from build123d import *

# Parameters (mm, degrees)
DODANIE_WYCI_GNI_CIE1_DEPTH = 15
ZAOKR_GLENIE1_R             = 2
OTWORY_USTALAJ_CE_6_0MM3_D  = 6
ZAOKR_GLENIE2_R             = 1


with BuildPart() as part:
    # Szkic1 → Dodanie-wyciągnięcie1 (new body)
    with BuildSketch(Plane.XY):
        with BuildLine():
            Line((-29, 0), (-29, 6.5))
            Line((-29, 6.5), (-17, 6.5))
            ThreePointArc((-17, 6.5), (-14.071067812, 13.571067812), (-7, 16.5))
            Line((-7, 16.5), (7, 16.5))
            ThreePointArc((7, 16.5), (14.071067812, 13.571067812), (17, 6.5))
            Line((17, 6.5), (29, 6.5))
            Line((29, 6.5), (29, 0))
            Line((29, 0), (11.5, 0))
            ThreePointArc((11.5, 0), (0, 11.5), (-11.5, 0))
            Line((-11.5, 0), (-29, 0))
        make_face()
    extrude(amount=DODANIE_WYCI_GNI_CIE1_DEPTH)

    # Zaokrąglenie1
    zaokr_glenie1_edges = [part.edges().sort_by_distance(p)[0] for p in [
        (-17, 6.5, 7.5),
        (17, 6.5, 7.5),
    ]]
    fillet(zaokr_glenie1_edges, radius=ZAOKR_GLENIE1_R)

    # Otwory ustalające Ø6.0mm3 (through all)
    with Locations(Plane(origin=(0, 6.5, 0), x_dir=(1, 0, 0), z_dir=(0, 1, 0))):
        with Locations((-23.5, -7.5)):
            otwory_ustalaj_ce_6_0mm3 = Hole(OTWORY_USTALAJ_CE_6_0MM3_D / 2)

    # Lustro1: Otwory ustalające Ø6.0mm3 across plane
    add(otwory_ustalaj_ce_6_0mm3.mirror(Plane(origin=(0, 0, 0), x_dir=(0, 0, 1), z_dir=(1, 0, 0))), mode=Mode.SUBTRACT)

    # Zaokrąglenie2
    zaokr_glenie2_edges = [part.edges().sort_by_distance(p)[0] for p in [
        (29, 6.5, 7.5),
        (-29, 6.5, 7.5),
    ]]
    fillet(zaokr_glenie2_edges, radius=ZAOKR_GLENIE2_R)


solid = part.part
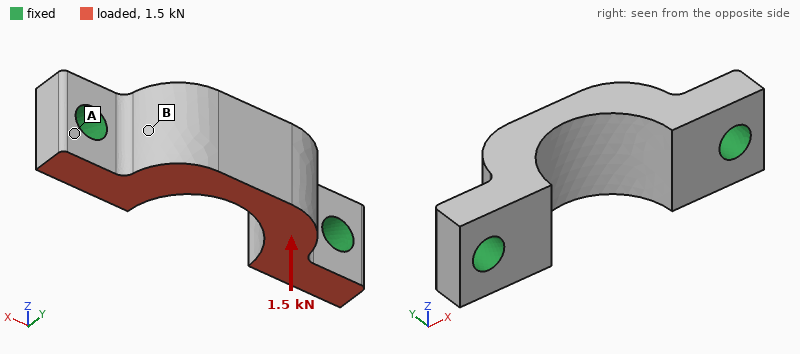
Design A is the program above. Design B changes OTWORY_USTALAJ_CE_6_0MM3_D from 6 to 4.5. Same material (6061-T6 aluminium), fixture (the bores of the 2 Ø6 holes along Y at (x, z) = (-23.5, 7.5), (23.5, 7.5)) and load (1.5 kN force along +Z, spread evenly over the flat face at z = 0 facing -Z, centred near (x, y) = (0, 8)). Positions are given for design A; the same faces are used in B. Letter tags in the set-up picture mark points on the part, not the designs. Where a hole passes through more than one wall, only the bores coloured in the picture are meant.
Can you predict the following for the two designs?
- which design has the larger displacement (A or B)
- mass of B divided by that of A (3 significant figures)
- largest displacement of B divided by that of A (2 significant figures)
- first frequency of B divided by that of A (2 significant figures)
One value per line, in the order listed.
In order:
B
1.02
1.3
0.88
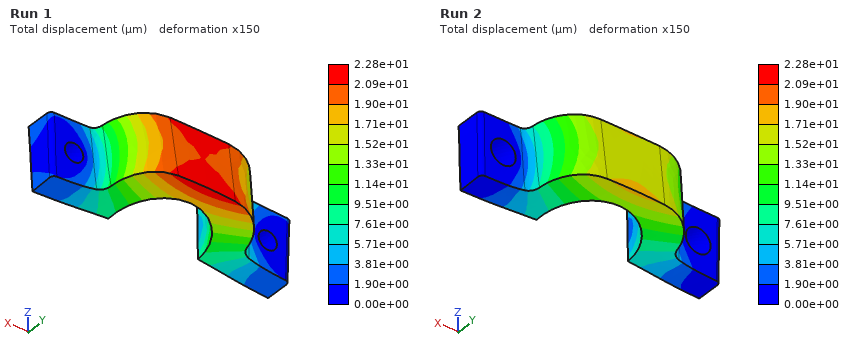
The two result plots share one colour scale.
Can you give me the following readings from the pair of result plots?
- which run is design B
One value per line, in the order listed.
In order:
Run 1
